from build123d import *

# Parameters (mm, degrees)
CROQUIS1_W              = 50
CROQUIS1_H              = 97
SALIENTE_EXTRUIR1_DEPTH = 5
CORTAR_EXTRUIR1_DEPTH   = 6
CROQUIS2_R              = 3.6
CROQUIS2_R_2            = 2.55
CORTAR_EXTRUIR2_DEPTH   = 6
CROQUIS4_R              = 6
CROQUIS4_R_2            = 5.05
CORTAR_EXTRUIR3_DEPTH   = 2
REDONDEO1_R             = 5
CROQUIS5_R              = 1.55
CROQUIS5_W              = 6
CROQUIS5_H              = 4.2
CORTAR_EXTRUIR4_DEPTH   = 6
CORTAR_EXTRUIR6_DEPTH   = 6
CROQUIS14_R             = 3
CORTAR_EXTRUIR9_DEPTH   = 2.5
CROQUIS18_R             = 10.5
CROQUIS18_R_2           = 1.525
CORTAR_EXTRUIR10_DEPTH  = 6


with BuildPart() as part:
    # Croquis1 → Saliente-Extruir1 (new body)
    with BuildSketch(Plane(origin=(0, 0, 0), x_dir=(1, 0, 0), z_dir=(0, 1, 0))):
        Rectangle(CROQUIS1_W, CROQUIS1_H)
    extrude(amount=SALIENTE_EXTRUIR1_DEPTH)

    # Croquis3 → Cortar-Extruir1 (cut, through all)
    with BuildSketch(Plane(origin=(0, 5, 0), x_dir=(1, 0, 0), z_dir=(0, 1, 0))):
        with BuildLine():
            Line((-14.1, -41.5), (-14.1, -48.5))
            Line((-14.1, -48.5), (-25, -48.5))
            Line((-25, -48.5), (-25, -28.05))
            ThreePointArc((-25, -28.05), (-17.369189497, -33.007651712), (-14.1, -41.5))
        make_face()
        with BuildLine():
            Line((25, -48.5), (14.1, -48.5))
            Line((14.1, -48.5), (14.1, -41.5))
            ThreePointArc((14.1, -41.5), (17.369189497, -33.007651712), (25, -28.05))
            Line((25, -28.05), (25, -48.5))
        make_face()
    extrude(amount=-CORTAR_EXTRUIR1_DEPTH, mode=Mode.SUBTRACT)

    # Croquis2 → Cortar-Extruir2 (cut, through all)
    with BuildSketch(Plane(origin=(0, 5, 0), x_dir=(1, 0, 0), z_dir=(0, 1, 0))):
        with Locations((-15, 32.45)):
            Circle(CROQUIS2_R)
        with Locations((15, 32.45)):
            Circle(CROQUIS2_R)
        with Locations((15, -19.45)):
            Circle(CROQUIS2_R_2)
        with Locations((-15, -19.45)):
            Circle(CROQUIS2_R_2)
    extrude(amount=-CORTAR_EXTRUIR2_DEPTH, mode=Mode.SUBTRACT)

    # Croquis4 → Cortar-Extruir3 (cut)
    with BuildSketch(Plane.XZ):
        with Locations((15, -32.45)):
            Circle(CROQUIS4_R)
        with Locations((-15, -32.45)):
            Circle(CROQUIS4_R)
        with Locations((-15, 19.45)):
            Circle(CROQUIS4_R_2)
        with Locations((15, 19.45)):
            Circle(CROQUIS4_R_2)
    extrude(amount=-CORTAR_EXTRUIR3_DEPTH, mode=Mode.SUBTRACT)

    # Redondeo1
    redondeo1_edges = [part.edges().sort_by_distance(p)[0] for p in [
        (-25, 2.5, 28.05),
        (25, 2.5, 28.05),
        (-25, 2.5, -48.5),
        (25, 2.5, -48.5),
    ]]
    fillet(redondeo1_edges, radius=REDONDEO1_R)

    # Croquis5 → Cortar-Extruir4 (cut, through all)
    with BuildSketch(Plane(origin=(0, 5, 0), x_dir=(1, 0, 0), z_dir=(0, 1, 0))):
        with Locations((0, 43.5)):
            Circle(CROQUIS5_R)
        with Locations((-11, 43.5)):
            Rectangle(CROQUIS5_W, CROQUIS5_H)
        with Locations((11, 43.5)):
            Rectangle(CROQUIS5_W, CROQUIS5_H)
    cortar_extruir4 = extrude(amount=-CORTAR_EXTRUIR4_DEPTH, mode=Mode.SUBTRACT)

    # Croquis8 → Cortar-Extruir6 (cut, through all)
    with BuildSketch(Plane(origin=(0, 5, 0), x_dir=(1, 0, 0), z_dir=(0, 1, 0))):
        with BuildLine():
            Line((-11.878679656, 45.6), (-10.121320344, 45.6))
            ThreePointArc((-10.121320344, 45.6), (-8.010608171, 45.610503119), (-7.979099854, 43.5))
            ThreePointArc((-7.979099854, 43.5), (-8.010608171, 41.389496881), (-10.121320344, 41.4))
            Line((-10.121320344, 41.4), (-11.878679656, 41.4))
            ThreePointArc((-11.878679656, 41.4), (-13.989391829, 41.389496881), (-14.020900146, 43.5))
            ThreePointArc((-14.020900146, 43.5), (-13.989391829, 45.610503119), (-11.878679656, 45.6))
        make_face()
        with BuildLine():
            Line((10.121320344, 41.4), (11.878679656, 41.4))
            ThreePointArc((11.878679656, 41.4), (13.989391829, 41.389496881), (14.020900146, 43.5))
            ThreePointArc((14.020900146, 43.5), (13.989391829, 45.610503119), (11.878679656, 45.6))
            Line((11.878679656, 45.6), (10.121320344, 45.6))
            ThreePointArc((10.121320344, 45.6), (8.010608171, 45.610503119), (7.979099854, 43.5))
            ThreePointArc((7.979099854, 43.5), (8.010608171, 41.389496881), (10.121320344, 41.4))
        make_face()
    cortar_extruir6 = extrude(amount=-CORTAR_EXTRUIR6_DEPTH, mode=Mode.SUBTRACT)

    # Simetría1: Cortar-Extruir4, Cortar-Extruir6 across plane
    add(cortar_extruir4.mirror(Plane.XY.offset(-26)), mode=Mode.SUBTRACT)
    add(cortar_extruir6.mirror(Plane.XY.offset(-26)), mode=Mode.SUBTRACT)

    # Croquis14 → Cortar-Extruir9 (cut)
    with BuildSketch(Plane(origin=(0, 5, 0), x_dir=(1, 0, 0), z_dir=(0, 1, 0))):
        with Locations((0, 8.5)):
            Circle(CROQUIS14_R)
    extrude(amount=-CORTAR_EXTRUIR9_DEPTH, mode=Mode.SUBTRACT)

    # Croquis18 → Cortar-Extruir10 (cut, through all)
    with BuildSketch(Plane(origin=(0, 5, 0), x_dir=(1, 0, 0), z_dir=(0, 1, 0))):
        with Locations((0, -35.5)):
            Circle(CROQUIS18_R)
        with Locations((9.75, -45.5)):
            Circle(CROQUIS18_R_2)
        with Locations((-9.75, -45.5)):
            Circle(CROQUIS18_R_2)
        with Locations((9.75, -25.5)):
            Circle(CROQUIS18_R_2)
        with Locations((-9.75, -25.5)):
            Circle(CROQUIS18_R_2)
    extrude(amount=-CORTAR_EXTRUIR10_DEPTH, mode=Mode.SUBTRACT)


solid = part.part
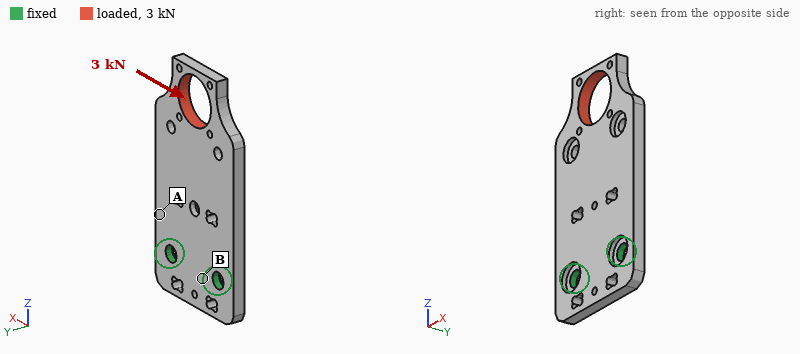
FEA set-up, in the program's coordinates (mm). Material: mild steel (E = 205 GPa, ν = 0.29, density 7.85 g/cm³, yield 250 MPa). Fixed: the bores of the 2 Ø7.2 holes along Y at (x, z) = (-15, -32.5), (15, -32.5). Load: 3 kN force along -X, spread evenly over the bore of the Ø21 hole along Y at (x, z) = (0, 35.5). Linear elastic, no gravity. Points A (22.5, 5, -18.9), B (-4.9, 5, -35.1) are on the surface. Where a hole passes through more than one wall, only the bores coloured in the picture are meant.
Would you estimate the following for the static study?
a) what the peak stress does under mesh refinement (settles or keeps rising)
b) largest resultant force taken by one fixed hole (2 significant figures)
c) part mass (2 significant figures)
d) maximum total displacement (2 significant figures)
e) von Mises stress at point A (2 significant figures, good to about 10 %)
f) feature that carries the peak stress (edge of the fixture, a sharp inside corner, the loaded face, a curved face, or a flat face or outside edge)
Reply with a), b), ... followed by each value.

a) keeps rising
b) 6.2 kN
c) 150 g
d) 90 µm
e) 86 MPa
f) edge of the fixture
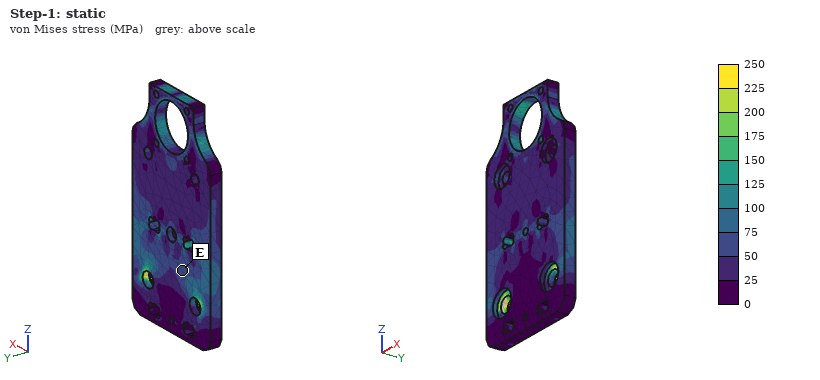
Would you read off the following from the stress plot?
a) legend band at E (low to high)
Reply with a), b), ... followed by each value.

a) 50 to 75 MPa
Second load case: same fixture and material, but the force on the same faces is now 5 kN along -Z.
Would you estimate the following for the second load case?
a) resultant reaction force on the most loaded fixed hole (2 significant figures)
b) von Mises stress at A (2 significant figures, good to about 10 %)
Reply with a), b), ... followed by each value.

a) 2.5 kN
b) 24 MPa
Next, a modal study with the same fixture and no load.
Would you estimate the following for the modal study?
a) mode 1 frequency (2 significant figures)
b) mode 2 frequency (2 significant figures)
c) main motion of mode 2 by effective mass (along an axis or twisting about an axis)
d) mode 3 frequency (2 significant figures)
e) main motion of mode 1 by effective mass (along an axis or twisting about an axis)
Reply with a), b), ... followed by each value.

a) 800 Hz
b) 2700 Hz
c) twisting about Z
d) 3900 Hz
e) along Y
